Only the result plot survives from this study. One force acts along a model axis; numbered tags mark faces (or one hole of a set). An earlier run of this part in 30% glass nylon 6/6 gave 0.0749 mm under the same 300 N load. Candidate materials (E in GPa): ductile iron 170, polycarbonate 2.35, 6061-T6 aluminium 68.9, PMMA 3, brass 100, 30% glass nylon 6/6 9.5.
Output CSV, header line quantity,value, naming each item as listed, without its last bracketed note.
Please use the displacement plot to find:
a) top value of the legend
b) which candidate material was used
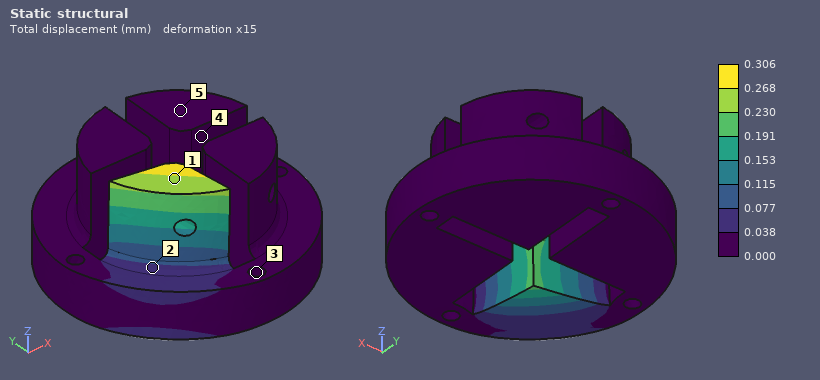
quantity,value
top value of the legend,0.306 mm
which candidate material was used,polycarbonate
